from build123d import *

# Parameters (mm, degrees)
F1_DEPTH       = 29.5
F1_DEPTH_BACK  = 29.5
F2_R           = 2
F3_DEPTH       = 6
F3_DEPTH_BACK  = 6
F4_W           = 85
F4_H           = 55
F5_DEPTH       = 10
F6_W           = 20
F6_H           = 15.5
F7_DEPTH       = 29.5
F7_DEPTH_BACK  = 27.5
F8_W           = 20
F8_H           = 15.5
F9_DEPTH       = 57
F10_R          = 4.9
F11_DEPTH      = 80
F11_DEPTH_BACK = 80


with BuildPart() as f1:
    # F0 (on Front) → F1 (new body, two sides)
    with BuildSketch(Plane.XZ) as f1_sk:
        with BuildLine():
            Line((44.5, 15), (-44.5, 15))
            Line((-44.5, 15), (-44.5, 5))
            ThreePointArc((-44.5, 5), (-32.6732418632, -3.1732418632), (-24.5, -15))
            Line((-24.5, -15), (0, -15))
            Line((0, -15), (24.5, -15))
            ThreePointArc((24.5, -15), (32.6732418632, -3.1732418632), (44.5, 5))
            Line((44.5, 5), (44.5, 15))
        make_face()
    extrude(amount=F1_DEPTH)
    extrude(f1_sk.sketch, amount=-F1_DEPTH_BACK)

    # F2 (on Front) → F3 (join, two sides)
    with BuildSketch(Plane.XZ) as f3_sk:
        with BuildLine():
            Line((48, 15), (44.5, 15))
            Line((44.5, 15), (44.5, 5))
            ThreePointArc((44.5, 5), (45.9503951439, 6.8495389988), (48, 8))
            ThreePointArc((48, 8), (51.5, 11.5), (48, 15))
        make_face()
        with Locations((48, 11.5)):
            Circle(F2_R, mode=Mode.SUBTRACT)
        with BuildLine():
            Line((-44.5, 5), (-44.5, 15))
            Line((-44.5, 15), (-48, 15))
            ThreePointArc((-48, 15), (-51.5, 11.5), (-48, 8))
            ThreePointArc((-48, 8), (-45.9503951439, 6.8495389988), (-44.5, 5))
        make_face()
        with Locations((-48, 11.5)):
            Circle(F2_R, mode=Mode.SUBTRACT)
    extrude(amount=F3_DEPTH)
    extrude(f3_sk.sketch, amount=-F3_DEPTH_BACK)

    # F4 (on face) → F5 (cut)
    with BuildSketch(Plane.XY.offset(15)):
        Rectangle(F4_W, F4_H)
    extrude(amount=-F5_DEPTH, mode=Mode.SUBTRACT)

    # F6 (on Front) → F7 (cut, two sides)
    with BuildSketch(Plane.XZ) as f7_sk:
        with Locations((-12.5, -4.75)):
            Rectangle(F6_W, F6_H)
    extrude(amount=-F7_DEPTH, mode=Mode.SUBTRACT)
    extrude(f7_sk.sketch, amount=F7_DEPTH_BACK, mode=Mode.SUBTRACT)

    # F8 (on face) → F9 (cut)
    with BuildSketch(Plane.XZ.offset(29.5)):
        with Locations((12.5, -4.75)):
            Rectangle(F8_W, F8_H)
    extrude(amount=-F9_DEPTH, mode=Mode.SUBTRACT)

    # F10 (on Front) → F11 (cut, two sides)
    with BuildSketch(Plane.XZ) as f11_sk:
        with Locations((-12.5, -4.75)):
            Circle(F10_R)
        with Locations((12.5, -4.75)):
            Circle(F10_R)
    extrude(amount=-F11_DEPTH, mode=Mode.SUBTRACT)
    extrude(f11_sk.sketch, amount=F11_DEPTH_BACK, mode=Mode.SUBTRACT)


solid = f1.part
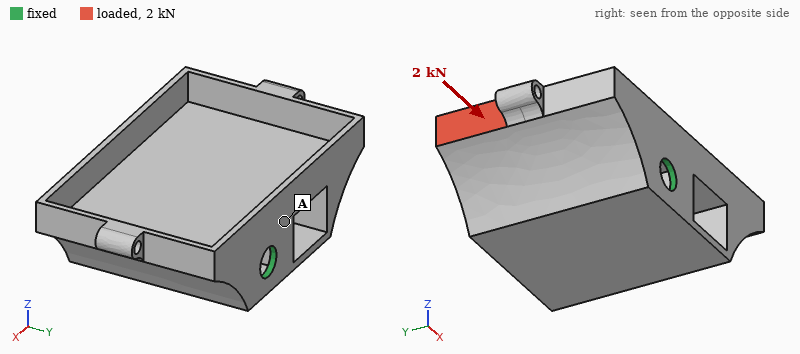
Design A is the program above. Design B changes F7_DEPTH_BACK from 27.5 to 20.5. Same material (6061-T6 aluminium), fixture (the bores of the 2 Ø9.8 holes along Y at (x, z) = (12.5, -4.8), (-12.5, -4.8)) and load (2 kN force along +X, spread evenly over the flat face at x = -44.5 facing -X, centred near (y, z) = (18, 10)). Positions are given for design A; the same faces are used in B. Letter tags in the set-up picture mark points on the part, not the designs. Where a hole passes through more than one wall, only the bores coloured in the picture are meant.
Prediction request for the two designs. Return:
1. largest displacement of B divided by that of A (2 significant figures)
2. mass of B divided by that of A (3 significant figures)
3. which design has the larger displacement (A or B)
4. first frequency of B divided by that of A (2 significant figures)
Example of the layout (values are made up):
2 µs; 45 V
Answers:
0.92; 1.04; A; 1.3
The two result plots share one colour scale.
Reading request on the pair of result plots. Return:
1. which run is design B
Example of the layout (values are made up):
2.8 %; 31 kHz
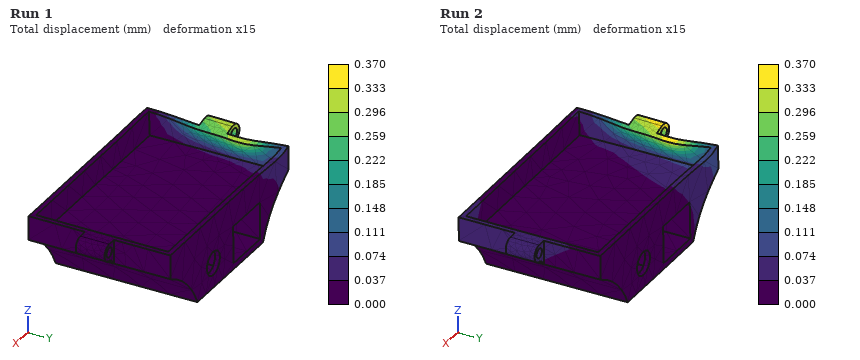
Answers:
Run 1
